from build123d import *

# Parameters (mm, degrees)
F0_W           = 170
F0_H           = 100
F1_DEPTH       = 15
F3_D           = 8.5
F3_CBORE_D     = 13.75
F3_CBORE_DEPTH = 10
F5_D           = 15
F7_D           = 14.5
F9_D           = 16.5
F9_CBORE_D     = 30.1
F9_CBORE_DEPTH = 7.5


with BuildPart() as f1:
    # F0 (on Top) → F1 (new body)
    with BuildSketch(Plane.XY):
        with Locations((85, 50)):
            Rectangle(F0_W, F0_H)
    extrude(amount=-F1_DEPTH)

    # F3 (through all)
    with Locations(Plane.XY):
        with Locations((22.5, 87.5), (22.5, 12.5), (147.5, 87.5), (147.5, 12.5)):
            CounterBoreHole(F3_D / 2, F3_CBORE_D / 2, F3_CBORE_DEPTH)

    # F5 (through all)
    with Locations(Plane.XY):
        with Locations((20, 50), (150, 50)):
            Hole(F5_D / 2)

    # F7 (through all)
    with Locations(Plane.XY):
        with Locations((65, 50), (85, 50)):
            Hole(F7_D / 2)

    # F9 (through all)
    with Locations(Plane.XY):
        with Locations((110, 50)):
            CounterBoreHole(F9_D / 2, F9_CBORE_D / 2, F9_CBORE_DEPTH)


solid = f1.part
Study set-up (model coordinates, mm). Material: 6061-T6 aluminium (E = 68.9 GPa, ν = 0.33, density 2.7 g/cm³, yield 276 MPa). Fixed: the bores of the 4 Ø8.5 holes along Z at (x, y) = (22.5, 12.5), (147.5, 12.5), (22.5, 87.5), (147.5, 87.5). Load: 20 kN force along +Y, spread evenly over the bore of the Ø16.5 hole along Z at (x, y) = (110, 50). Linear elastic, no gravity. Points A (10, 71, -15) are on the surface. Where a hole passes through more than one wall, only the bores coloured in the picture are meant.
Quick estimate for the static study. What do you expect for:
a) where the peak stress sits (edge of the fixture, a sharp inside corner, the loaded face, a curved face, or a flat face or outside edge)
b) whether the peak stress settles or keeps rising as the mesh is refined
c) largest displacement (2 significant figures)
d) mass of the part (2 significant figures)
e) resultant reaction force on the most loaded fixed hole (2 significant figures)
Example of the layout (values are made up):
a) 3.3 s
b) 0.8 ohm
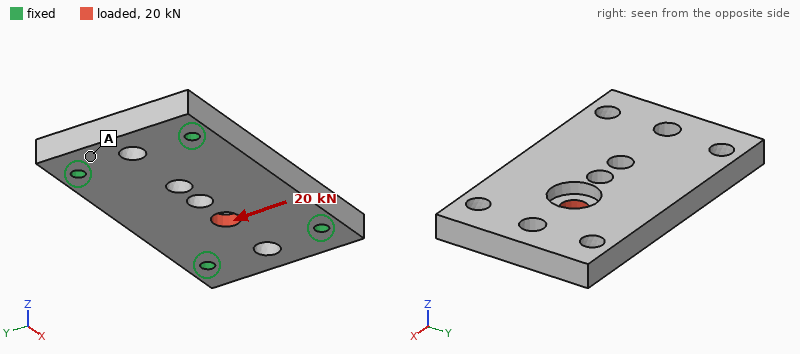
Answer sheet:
a) edge of the fixture
b) keeps rising
c) 37 µm
d) 620 g
e) 7.4 kN
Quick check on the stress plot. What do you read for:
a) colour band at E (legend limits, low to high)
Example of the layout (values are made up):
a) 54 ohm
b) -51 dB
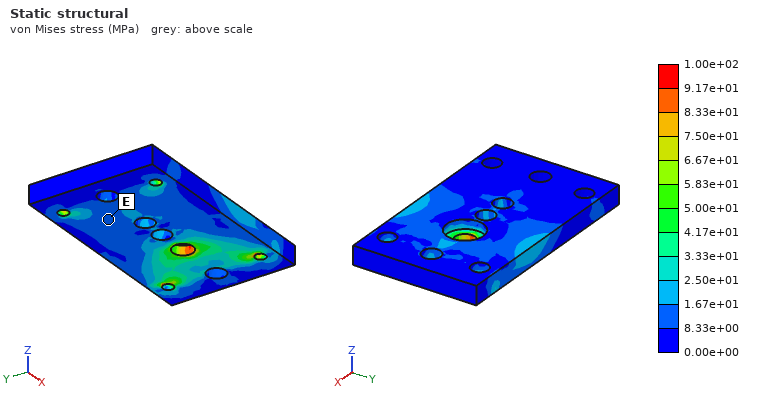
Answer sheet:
a) 8.33e+00 to 1.67e+01 MPa
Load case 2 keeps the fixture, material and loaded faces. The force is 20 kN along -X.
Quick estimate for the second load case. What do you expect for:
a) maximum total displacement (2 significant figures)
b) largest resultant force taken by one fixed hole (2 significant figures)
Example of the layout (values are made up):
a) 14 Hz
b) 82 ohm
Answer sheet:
a) 32 µm
b) 6.4 kN
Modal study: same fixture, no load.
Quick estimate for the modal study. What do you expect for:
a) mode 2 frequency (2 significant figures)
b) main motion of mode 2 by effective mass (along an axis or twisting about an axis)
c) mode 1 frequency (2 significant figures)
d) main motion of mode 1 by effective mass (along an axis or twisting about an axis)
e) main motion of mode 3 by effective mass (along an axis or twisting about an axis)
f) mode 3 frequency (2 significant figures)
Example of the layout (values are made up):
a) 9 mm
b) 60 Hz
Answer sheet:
a) 4700 Hz
b) twisting about X
c) 3000 Hz
d) along Z
e) along Z
f) 6800 Hz
